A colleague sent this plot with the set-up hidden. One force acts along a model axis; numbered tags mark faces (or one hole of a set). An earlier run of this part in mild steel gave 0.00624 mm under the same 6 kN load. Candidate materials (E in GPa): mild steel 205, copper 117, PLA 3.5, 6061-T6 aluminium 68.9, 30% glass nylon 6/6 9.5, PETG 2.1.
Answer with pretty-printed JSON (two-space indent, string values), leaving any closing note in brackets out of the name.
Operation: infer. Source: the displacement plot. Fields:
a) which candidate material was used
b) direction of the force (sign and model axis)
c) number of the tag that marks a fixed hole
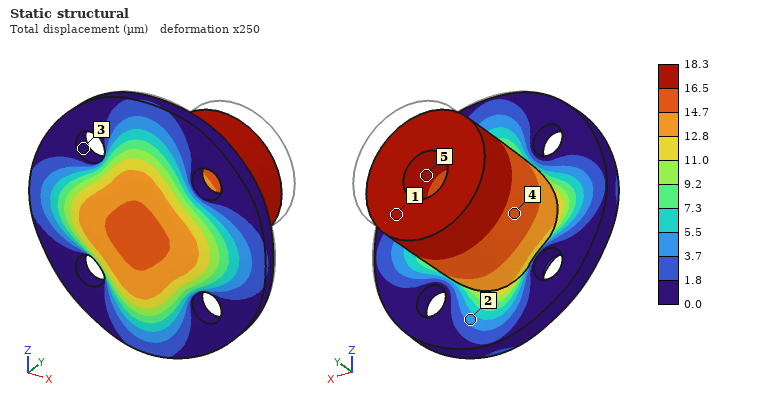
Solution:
{
  "which candidate material was used": "6061-T6 aluminium",
  "direction of the force": "-Y",
  "number of the tag that marks a fixed hole": "3"
}
